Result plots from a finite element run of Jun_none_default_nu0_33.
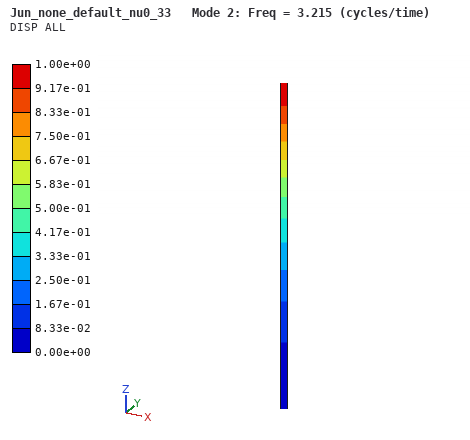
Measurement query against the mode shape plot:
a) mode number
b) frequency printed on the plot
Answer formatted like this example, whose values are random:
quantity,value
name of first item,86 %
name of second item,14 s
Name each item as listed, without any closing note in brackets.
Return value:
quantity,value
mode number,2
frequency printed on the plot,3.215
